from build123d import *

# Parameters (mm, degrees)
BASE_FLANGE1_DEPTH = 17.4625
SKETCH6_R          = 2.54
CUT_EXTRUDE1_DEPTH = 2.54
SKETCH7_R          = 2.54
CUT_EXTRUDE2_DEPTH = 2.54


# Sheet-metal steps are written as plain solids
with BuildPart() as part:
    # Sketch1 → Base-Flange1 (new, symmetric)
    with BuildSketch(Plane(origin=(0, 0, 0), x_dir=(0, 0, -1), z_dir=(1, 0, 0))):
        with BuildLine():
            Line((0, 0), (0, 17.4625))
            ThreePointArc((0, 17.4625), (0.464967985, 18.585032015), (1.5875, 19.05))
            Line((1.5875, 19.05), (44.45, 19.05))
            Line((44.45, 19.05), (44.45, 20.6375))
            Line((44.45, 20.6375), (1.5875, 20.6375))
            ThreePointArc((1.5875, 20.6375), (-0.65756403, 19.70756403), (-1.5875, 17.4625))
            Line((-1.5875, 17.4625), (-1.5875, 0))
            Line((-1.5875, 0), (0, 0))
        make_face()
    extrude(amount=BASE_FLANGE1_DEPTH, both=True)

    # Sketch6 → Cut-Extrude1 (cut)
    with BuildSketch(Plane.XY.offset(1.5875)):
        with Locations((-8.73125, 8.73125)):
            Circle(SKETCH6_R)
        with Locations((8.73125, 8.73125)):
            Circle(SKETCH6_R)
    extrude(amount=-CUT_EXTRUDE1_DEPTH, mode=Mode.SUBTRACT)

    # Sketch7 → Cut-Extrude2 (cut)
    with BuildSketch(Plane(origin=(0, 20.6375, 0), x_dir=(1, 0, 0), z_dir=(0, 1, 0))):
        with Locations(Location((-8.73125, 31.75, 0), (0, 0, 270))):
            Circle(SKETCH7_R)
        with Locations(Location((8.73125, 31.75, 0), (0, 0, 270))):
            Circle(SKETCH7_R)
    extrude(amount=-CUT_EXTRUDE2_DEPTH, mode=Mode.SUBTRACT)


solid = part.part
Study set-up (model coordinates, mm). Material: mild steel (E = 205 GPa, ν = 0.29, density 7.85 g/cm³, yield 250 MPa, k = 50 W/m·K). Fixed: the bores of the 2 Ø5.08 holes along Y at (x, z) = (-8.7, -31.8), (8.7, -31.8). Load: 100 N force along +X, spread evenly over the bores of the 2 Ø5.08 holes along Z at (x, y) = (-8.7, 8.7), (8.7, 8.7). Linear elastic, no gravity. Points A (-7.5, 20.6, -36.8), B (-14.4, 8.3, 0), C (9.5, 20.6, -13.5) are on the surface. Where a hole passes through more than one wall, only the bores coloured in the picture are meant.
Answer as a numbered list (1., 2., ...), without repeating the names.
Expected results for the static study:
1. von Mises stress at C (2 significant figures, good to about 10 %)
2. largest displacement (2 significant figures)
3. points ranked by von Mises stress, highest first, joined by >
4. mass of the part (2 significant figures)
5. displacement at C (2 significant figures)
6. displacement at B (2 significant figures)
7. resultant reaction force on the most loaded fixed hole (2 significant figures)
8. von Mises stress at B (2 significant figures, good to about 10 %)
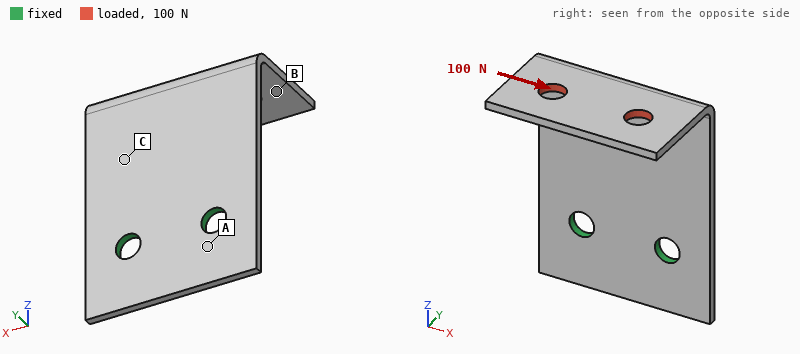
1. 48 MPa
2. 0.17 mm
3. C > B > A
4. 27 g
5. 0.028 mm
6. 0.12 mm
7. 170 N
8. 16 MPa
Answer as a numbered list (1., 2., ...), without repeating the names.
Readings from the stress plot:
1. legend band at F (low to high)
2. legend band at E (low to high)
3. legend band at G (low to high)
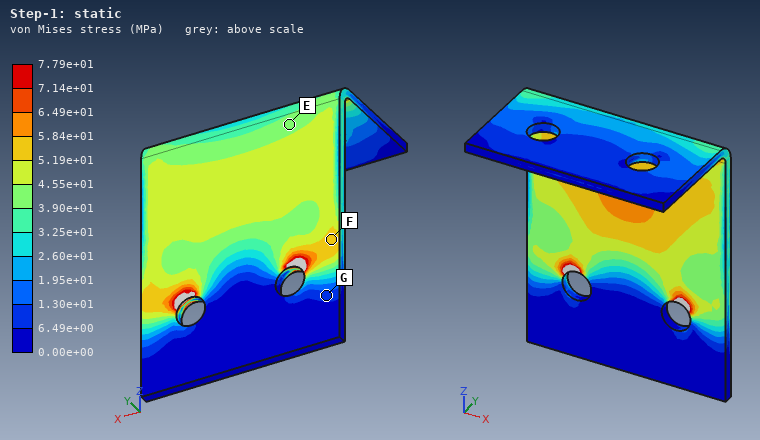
1. 5.19e+01 to 5.84e+01 MPa
2. 3.90e+01 to 4.55e+01 MPa
3. 6.49e+00 to 1.30e+01 MPa
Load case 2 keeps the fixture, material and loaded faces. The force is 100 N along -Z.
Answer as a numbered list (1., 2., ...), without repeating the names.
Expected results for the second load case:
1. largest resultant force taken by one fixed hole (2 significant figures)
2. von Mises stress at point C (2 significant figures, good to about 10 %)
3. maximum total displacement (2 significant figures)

1. 51 N
2. 68 MPa
3. 0.38 mm
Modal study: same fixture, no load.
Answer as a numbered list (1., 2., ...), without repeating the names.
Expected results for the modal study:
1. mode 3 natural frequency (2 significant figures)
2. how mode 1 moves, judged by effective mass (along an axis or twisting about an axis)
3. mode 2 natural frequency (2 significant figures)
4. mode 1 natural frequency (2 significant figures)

1. 2300 Hz
2. along Y
3. 1400 Hz
4. 680 Hz
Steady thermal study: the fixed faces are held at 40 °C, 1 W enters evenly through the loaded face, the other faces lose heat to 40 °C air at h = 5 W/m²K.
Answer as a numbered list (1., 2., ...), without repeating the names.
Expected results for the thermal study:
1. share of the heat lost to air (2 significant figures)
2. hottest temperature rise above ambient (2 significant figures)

1. 15 %
2. 15 K
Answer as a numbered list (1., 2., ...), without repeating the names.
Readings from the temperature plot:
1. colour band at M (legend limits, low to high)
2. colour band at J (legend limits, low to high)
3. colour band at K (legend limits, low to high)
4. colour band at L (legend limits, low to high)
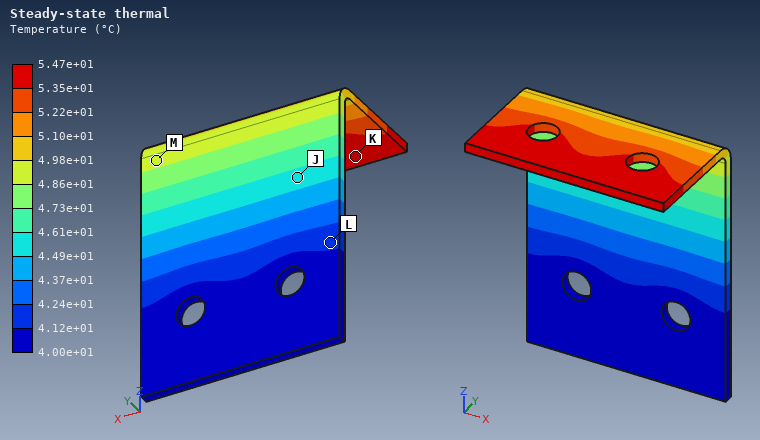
1. 4.86e+01 to 4.98e+01 °C
2. 4.49e+01 to 4.61e+01 °C
3. 5.35e+01 to 5.47e+01 °C
4. 4.12e+01 to 4.24e+01 °C
